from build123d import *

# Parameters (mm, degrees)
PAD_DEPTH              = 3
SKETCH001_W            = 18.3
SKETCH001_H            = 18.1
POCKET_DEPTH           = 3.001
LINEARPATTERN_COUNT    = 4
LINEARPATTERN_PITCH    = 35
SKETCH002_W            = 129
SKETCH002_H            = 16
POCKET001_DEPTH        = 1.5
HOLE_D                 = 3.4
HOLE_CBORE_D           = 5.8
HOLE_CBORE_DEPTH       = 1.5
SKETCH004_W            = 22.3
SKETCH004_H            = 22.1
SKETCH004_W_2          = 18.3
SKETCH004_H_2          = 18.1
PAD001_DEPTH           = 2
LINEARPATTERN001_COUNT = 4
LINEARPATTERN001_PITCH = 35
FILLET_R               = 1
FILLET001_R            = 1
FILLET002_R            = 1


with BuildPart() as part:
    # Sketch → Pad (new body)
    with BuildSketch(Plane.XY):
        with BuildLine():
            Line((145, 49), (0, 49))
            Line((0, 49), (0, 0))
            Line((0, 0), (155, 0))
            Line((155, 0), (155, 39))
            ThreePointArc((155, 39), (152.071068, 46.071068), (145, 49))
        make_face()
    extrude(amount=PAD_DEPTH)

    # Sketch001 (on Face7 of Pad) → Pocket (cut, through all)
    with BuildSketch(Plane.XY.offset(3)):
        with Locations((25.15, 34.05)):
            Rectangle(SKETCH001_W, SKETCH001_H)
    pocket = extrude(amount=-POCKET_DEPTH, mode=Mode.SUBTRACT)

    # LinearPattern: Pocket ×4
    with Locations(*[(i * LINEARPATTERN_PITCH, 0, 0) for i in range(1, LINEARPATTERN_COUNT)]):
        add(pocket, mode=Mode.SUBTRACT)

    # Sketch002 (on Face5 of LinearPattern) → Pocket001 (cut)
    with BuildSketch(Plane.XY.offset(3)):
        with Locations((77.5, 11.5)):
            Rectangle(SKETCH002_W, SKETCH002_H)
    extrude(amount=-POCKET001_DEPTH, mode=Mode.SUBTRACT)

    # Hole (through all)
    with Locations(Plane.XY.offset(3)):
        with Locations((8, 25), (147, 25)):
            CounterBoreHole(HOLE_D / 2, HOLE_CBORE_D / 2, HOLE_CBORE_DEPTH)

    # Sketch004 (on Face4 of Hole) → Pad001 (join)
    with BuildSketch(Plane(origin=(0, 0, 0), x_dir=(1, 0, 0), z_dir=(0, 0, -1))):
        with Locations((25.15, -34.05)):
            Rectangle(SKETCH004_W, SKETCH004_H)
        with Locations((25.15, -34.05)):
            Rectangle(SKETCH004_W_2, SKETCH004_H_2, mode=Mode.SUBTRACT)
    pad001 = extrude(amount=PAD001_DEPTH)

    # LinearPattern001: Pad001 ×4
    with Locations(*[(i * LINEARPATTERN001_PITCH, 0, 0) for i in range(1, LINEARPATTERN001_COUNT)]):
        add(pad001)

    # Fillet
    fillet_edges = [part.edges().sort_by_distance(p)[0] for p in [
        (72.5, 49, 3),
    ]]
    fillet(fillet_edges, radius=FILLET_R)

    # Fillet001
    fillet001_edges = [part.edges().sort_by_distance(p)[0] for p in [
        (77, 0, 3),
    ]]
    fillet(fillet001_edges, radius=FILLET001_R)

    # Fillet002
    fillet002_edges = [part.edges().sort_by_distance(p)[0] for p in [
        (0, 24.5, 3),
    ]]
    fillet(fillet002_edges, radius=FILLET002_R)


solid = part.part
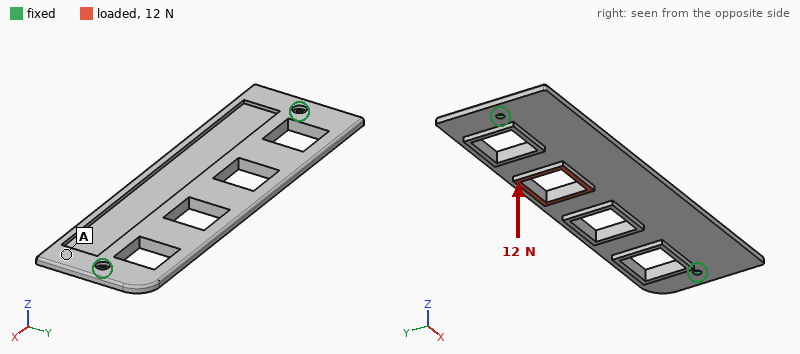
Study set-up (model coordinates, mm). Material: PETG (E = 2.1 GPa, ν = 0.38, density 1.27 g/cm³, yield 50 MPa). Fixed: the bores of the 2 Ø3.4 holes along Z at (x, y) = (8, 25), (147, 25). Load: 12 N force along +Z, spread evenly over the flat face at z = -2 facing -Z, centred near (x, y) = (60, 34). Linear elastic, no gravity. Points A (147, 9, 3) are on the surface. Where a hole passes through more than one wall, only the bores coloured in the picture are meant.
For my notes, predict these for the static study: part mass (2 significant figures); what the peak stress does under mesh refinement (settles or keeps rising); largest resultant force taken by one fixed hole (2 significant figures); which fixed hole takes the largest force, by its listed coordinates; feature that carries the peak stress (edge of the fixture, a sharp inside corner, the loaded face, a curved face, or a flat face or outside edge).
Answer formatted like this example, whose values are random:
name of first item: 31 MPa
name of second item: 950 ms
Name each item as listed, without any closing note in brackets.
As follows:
part mass: 21 g
what the peak stress does under mesh refinement: keeps rising
largest resultant force taken by one fixed hole: 9.6 N
which fixed hole takes the largest force, by its listed coordinates: (8, 25)
feature that carries the peak stress: edge of the fixture
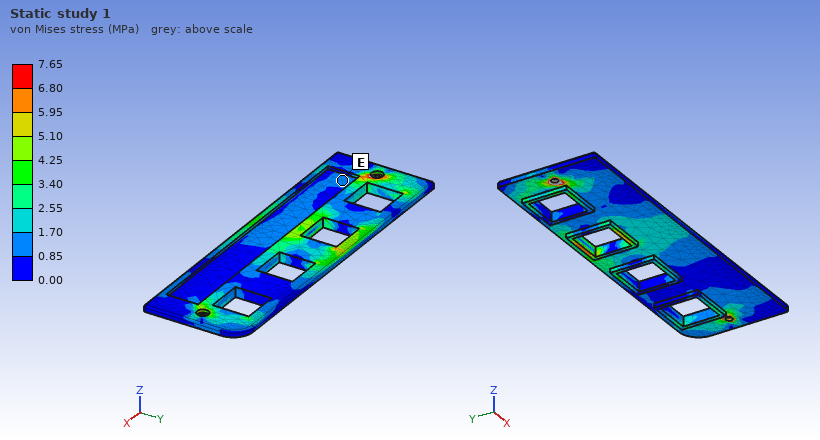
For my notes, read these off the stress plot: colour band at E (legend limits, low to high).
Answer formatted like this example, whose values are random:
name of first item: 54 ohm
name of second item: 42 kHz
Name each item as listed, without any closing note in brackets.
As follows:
colour band at E: 0.85 to 1.70 MPa
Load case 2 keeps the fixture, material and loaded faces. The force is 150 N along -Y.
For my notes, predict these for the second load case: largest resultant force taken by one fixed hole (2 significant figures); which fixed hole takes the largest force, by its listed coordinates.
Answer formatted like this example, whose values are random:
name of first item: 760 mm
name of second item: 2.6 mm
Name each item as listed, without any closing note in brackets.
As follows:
largest resultant force taken by one fixed hole: 100 N
which fixed hole takes the largest force, by its listed coordinates: (8, 25)
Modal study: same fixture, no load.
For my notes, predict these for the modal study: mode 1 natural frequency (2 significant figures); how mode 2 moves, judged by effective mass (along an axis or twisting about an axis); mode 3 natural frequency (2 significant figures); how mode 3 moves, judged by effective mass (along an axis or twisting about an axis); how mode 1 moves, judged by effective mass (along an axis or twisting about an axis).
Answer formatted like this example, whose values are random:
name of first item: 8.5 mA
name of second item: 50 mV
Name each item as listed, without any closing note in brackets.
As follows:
mode 1 natural frequency: 160 Hz
how mode 2 moves, judged by effective mass: twisting about X
mode 3 natural frequency: 440 Hz
how mode 3 moves, judged by effective mass: twisting about Y
how mode 1 moves, judged by effective mass: along Z
